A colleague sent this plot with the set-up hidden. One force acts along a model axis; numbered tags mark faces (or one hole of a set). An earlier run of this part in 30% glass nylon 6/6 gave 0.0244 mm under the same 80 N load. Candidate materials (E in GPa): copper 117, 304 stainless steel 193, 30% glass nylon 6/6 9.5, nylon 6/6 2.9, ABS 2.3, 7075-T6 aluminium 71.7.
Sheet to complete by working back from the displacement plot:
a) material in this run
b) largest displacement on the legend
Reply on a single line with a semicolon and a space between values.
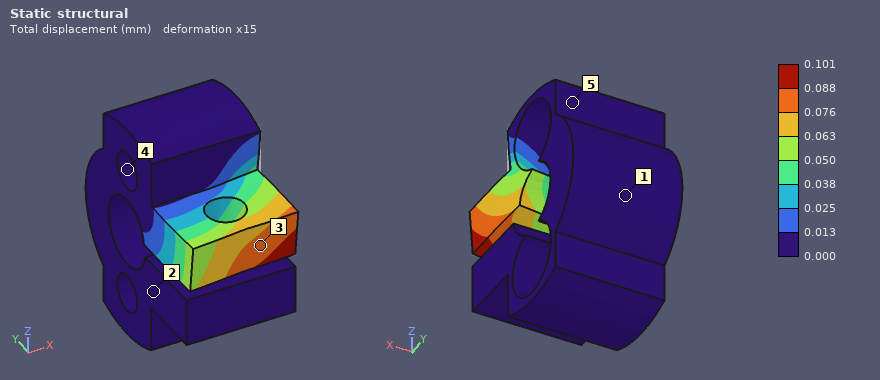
ABS; 0.101 mm
